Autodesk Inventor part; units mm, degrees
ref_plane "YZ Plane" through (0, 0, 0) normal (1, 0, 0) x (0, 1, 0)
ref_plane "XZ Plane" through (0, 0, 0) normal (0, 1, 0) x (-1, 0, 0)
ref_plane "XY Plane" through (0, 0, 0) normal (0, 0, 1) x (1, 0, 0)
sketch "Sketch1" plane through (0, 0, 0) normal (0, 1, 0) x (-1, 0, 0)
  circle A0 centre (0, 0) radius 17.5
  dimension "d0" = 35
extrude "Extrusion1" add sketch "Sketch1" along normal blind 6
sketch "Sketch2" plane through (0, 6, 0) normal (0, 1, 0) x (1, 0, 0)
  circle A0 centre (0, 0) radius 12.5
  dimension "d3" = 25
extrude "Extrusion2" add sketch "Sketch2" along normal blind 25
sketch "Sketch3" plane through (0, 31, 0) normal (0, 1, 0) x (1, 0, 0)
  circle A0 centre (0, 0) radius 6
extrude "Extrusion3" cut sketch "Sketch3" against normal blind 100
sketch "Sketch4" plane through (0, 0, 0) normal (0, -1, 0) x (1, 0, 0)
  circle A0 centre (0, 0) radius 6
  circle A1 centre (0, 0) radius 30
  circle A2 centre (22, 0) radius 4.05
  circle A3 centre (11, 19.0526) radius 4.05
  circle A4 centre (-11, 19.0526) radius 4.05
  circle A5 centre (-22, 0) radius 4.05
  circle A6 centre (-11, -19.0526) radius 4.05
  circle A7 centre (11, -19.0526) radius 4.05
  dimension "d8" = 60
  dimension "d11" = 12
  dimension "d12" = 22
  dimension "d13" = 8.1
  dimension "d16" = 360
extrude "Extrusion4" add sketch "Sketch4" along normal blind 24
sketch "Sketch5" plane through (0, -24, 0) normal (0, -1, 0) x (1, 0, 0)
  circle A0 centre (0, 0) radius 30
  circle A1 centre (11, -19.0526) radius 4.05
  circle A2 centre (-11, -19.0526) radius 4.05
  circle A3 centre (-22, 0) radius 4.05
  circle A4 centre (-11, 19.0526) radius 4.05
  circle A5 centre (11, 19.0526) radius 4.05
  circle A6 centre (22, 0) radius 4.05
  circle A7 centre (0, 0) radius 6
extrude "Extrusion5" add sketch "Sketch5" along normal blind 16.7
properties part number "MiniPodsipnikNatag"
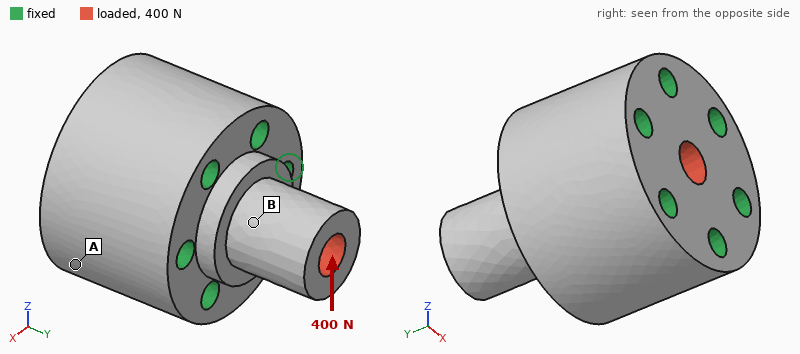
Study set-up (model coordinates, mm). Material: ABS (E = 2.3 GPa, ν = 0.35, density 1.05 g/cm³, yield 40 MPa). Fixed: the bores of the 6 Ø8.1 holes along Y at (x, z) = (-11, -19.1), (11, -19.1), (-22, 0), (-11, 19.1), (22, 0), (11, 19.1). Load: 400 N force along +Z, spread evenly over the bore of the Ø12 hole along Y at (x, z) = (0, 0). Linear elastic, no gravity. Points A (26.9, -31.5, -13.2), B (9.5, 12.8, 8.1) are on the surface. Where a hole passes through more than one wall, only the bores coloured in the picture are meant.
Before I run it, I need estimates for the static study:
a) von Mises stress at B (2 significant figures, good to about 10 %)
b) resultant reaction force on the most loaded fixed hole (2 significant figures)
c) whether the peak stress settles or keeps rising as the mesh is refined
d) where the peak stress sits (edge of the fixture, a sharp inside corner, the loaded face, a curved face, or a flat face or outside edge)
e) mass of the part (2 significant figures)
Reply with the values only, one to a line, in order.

0.61 MPa
120 N
keeps rising
edge of the fixture
120 g
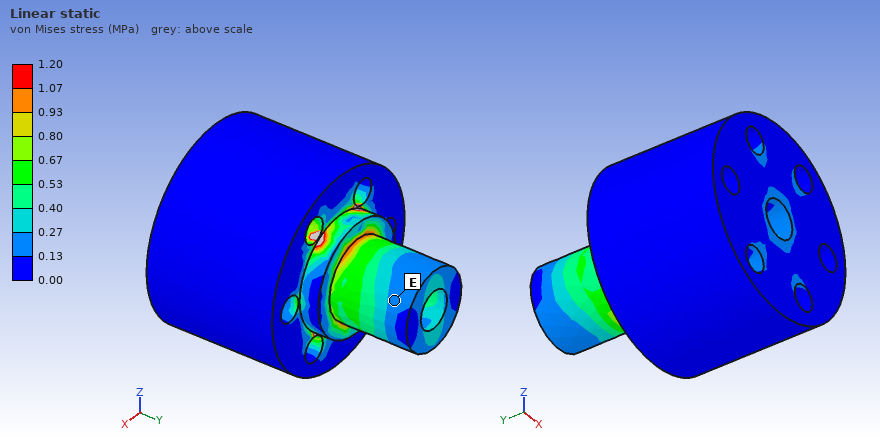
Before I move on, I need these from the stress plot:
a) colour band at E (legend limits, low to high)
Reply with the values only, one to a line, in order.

0.13 to 0.27 MPa
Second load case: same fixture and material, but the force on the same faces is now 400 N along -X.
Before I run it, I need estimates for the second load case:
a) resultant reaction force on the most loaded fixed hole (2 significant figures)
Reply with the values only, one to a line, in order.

130 N
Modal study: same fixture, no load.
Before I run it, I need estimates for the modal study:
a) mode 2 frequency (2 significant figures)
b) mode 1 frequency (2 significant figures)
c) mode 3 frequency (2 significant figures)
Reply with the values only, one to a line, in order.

4500 Hz
4500 Hz
7700 Hz
